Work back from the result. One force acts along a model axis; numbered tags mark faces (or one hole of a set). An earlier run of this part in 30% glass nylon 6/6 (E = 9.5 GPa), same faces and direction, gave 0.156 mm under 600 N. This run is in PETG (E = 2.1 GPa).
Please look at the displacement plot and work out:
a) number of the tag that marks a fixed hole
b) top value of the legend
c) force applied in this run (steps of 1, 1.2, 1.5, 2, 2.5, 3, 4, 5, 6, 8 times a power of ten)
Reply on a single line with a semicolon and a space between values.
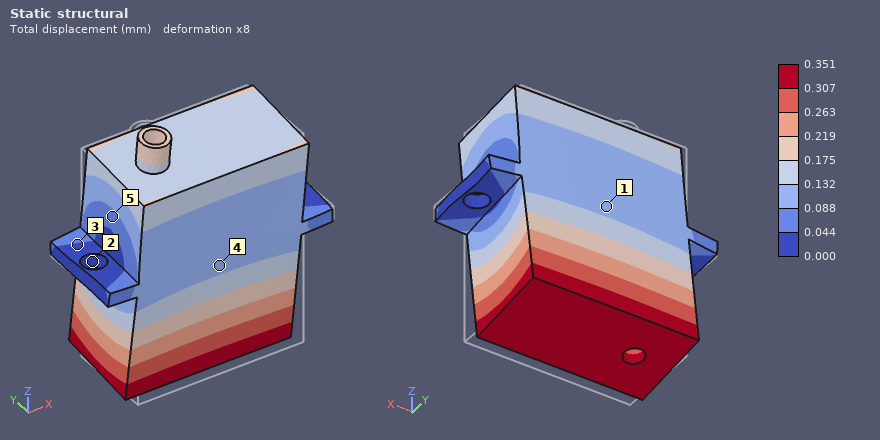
2; 0.351 mm; 300 N
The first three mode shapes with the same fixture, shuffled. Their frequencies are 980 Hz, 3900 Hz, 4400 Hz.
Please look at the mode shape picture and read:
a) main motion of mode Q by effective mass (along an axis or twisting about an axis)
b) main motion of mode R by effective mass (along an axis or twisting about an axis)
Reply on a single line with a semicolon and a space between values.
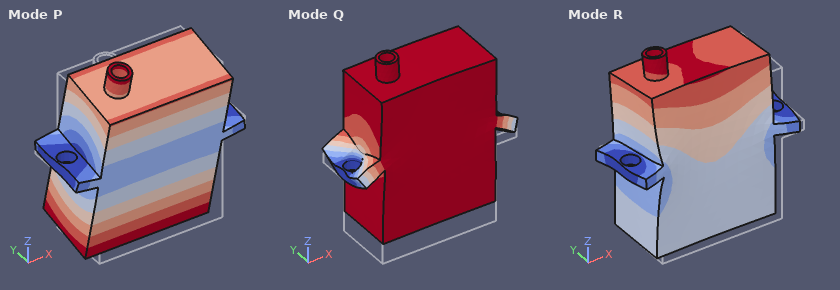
along Z; along Y
